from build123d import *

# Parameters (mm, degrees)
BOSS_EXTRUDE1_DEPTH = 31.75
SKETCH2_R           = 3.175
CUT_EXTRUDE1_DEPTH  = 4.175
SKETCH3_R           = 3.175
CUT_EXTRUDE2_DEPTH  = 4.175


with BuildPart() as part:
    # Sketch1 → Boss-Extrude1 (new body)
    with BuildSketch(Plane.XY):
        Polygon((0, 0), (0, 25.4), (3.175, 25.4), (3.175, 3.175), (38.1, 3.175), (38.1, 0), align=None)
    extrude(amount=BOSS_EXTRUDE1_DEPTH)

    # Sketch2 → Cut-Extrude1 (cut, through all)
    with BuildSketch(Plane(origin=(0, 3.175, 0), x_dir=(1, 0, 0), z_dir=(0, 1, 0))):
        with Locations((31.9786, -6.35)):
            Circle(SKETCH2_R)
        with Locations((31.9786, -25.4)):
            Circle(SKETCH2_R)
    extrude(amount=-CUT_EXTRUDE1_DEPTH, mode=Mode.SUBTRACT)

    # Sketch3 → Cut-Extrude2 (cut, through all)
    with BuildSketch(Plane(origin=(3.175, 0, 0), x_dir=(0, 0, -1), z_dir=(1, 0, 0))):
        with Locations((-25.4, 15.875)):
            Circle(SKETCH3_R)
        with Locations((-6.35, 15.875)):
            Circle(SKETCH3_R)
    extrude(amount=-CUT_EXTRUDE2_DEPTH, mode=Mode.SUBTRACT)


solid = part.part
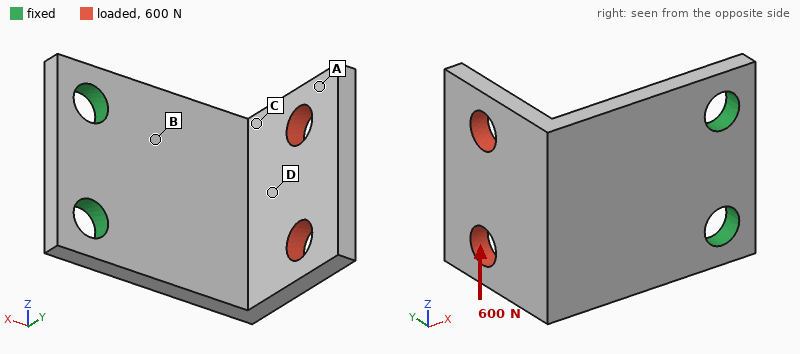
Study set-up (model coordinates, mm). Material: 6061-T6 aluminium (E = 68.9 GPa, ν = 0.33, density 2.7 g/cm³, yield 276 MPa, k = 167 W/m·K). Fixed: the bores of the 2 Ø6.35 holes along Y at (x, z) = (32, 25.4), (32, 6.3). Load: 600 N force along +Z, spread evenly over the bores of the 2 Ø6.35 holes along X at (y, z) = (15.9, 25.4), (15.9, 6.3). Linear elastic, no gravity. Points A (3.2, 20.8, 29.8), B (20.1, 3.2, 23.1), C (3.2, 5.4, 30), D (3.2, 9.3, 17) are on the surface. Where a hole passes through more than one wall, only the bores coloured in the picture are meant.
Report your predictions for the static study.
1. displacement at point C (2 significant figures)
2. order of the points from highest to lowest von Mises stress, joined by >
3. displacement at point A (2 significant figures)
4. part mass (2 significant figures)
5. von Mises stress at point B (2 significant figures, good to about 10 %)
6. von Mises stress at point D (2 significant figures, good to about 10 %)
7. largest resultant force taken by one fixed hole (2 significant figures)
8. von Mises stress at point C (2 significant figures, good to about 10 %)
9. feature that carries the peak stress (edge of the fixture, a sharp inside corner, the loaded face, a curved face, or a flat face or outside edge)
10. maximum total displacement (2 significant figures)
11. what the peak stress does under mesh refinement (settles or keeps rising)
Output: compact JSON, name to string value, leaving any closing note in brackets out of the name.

{"displacement at point C": "0.26 mm", "order of the points from highest to lowest von Mises stress, joined by >": "B > C > D > A", "displacement at point A": "0.44 mm", "part mass": "15 g", "von Mises stress at point B": "110 MPa", "von Mises stress at point D": "43 MPa", "largest resultant force taken by one fixed hole": "910 N", "von Mises stress at point C": "78 MPa", "feature that carries the peak stress": "edge of the fixture", "maximum total displacement": "0.53 mm", "what the peak stress does under mesh refinement": "keeps rising"}
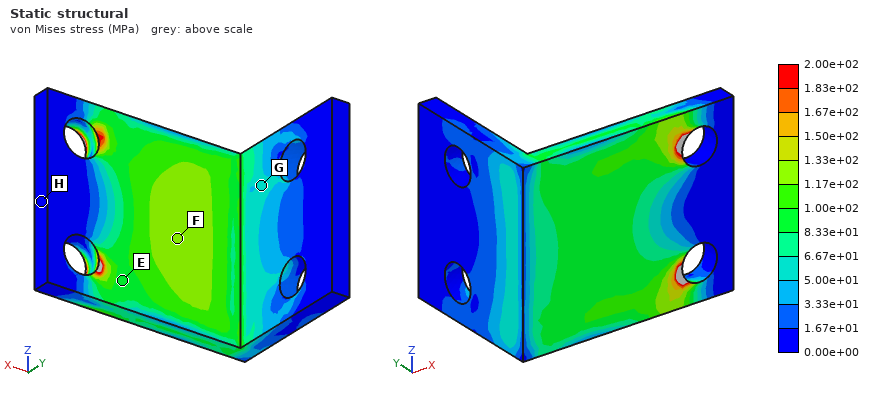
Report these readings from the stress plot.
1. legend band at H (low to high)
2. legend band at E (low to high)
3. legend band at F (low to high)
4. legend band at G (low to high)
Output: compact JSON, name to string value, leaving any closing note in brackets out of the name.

{"legend band at H": "0.00e+00 to 1.67e+01 MPa", "legend band at E": "8.33e+01 to 1.00e+02 MPa", "legend band at F": "1.17e+02 to 1.33e+02 MPa", "legend band at G": "5.00e+01 to 6.67e+01 MPa"}
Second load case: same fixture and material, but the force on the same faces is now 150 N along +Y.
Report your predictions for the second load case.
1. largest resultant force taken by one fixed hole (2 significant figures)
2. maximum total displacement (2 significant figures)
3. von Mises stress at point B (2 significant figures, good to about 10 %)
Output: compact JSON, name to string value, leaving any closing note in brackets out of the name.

{"largest resultant force taken by one fixed hole": "75 N", "maximum total displacement": "0.31 mm", "von Mises stress at point B": "47 MPa"}
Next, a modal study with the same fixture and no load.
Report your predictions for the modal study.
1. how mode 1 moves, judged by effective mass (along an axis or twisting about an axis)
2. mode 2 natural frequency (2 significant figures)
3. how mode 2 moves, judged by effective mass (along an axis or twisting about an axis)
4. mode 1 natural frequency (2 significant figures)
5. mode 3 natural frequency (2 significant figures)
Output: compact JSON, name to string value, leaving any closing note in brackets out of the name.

{"how mode 1 moves, judged by effective mass": "along Y", "mode 2 natural frequency": "2600 Hz", "how mode 2 moves, judged by effective mass": "along Z", "mode 1 natural frequency": "1300 Hz", "mode 3 natural frequency": "3900 Hz"}
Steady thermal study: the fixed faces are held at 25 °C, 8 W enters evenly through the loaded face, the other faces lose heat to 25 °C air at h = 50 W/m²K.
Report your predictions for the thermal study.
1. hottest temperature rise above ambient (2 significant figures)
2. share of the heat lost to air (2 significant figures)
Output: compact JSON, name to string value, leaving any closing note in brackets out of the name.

{"hottest temperature rise above ambient": "18 K", "share of the heat lost to air": "22 %"}
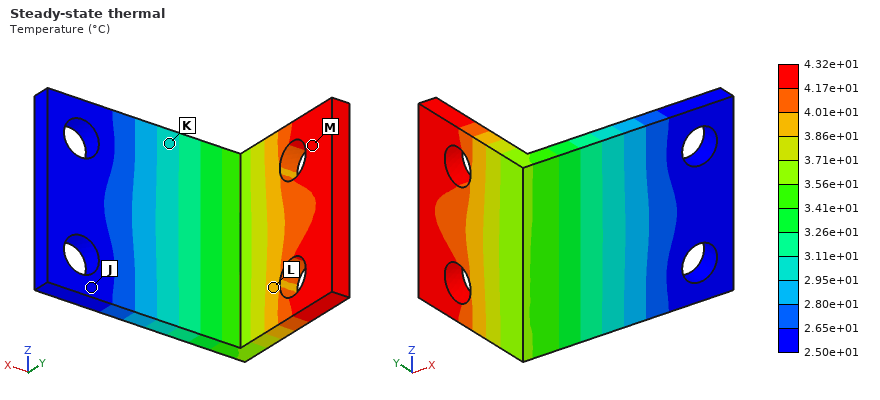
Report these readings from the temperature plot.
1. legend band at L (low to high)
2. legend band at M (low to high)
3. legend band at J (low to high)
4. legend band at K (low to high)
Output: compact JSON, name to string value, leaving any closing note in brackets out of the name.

{"legend band at L": "3.86e+01 to 4.01e+01 °C", "legend band at M": "4.17e+01 to 4.32e+01 °C", "legend band at J": "2.50e+01 to 2.65e+01 °C", "legend band at K": "2.95e+01 to 3.11e+01 °C"}
